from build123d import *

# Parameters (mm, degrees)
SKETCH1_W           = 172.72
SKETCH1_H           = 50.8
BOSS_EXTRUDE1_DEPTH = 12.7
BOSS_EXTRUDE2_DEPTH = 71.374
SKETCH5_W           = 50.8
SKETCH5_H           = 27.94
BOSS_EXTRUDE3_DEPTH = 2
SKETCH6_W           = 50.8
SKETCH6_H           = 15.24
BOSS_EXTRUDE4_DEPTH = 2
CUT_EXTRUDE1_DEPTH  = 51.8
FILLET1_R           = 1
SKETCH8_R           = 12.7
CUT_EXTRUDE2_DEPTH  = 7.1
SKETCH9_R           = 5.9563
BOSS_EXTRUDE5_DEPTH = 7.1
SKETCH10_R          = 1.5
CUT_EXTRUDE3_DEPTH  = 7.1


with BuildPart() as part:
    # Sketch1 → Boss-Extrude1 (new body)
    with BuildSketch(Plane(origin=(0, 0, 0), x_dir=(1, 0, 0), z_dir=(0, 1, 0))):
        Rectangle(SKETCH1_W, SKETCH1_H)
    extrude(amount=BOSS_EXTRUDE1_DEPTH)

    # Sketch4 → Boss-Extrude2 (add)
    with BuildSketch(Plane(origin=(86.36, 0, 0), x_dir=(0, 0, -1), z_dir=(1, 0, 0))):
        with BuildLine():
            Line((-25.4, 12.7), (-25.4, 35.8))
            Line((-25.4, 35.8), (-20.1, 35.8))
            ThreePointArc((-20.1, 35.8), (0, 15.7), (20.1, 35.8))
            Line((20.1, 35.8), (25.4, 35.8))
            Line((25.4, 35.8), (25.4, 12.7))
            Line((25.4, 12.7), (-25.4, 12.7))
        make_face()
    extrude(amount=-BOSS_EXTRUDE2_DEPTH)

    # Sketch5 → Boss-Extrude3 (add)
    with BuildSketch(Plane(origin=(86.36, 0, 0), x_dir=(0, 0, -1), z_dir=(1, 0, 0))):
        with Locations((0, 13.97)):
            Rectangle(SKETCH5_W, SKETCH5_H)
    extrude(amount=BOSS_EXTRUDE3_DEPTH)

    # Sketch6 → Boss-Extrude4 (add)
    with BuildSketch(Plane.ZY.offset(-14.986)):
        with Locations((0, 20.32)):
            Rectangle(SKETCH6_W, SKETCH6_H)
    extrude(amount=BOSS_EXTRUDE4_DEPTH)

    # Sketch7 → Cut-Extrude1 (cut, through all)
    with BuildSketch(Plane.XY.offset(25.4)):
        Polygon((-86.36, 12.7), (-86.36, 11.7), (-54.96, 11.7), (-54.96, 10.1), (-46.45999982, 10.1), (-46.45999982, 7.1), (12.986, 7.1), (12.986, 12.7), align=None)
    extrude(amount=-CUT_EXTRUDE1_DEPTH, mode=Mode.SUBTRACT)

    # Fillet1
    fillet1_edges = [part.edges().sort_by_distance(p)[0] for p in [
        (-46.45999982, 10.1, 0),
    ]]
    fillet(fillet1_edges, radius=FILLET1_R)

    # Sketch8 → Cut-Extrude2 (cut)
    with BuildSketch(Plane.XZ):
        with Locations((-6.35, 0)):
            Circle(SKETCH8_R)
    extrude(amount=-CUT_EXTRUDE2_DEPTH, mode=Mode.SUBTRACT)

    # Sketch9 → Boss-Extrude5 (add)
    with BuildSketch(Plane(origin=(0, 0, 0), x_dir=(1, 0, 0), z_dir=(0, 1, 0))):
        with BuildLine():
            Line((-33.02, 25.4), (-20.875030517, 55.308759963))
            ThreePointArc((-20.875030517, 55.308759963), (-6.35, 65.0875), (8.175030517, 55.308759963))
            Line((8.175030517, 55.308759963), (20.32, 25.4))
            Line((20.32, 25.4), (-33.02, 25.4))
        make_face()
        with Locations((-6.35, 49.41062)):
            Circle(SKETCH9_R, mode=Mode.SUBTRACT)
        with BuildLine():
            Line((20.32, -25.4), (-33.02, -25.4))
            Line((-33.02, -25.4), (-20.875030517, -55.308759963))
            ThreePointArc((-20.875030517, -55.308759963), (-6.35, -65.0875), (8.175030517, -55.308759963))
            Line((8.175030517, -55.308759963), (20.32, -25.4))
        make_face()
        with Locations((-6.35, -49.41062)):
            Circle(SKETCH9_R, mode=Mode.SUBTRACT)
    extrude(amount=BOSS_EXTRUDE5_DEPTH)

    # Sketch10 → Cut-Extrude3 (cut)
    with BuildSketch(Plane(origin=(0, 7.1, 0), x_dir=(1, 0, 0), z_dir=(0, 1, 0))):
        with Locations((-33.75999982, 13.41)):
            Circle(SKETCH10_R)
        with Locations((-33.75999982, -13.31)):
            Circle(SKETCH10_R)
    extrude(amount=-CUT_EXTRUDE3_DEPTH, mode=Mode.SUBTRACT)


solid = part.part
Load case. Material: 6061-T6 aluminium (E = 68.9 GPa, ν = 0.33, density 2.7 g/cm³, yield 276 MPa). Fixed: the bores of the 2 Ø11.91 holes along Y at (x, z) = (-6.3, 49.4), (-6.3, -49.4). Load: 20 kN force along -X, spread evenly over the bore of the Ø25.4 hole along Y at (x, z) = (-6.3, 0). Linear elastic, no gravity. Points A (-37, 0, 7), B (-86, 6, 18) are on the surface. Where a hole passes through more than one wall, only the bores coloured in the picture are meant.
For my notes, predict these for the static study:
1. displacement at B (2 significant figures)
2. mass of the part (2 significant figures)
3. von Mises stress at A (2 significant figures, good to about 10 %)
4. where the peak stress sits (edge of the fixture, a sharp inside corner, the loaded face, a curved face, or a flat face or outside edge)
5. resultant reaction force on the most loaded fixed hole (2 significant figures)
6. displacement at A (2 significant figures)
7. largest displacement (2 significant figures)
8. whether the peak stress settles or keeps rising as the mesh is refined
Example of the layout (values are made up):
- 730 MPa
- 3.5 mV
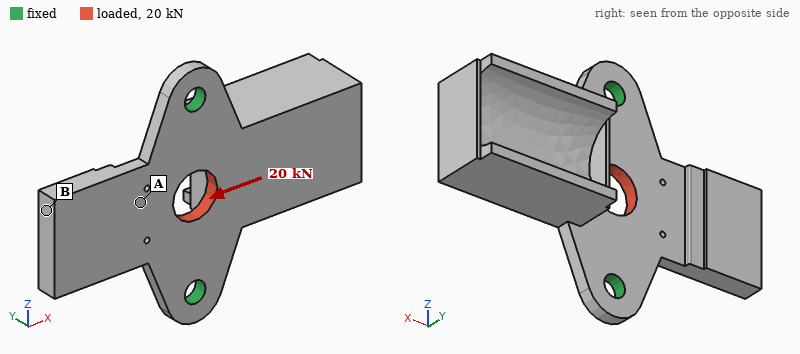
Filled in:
- 52 µm
- 400 g
- 32 MPa
- edge of the fixture
- 10 kN
- 51 µm
- 75 µm
- keeps rising
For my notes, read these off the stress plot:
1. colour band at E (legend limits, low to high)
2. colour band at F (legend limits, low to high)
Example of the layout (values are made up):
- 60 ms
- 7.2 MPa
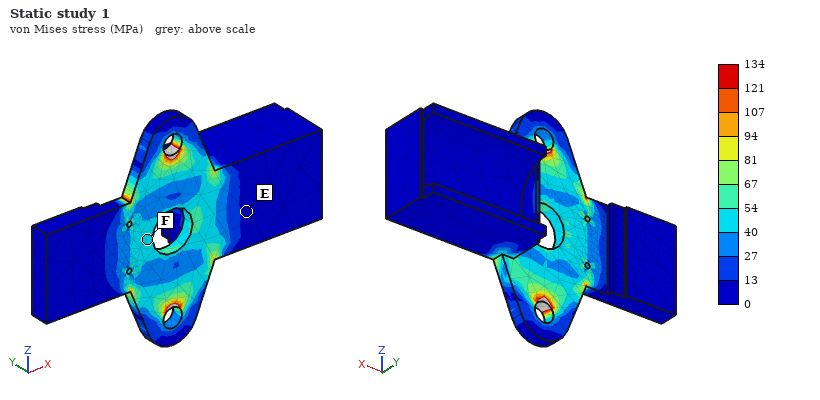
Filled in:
- 0 to 13 MPa
- 40 to 54 MPa
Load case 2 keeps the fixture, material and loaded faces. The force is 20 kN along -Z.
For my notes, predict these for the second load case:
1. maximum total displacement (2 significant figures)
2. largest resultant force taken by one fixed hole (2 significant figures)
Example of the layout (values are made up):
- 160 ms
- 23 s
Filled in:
- 27 µm
- 10 kN
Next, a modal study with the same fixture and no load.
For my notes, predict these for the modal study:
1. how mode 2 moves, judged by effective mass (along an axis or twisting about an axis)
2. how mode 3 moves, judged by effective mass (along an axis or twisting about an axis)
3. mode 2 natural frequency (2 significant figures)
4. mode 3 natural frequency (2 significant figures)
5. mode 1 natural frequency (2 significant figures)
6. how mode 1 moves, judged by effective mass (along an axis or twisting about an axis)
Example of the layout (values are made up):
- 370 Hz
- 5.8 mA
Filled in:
- along Y
- along Z
- 710 Hz
- 2500 Hz
- 410 Hz
- along Y
